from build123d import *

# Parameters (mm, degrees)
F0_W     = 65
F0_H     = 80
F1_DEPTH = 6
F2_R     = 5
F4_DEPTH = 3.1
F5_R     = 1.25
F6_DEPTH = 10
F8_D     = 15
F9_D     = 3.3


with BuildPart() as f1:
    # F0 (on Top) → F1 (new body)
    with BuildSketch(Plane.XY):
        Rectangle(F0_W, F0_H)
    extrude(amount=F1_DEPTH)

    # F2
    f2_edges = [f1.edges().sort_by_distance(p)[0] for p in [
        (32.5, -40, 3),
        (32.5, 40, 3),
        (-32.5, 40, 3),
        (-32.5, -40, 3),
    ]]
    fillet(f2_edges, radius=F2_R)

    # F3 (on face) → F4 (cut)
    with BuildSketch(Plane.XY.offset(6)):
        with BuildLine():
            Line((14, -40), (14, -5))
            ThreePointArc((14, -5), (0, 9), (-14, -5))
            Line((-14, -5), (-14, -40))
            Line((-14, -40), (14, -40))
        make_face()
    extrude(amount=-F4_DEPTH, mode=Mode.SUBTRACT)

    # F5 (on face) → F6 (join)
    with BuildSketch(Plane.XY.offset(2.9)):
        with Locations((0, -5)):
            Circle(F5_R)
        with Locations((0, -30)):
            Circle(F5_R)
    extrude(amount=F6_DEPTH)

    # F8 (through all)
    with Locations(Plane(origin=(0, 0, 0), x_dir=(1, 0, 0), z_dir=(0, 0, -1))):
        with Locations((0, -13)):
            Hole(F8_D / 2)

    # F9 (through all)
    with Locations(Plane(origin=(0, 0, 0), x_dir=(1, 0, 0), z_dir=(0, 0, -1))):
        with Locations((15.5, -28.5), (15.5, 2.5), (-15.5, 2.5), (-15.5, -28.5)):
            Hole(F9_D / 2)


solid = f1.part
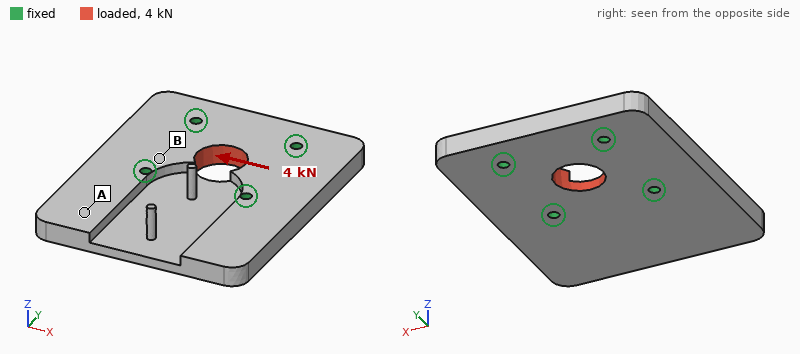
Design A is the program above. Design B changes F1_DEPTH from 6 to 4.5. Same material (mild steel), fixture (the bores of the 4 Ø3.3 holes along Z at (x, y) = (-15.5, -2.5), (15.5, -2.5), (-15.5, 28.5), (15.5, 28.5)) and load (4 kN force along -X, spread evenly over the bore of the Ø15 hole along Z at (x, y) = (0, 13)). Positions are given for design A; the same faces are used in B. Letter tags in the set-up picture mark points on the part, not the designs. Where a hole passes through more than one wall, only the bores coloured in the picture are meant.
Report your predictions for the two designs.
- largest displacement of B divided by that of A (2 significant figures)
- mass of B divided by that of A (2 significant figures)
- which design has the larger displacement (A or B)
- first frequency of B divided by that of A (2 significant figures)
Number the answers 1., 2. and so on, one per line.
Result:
1. 1.3
2. 0.79
3. B
4. 0.76
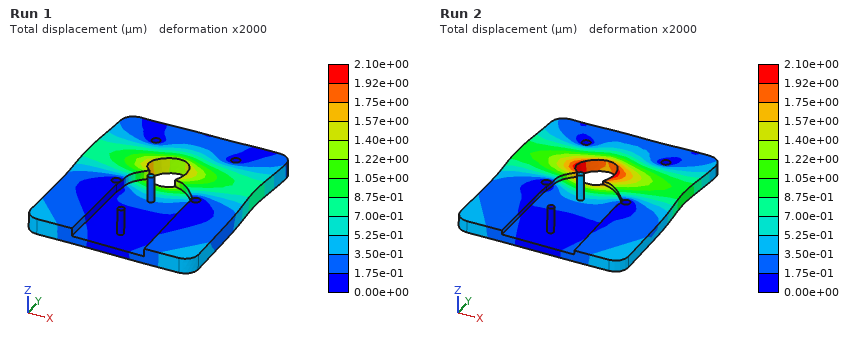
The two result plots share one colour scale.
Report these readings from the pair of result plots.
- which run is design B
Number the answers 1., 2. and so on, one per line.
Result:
1. Run 2
